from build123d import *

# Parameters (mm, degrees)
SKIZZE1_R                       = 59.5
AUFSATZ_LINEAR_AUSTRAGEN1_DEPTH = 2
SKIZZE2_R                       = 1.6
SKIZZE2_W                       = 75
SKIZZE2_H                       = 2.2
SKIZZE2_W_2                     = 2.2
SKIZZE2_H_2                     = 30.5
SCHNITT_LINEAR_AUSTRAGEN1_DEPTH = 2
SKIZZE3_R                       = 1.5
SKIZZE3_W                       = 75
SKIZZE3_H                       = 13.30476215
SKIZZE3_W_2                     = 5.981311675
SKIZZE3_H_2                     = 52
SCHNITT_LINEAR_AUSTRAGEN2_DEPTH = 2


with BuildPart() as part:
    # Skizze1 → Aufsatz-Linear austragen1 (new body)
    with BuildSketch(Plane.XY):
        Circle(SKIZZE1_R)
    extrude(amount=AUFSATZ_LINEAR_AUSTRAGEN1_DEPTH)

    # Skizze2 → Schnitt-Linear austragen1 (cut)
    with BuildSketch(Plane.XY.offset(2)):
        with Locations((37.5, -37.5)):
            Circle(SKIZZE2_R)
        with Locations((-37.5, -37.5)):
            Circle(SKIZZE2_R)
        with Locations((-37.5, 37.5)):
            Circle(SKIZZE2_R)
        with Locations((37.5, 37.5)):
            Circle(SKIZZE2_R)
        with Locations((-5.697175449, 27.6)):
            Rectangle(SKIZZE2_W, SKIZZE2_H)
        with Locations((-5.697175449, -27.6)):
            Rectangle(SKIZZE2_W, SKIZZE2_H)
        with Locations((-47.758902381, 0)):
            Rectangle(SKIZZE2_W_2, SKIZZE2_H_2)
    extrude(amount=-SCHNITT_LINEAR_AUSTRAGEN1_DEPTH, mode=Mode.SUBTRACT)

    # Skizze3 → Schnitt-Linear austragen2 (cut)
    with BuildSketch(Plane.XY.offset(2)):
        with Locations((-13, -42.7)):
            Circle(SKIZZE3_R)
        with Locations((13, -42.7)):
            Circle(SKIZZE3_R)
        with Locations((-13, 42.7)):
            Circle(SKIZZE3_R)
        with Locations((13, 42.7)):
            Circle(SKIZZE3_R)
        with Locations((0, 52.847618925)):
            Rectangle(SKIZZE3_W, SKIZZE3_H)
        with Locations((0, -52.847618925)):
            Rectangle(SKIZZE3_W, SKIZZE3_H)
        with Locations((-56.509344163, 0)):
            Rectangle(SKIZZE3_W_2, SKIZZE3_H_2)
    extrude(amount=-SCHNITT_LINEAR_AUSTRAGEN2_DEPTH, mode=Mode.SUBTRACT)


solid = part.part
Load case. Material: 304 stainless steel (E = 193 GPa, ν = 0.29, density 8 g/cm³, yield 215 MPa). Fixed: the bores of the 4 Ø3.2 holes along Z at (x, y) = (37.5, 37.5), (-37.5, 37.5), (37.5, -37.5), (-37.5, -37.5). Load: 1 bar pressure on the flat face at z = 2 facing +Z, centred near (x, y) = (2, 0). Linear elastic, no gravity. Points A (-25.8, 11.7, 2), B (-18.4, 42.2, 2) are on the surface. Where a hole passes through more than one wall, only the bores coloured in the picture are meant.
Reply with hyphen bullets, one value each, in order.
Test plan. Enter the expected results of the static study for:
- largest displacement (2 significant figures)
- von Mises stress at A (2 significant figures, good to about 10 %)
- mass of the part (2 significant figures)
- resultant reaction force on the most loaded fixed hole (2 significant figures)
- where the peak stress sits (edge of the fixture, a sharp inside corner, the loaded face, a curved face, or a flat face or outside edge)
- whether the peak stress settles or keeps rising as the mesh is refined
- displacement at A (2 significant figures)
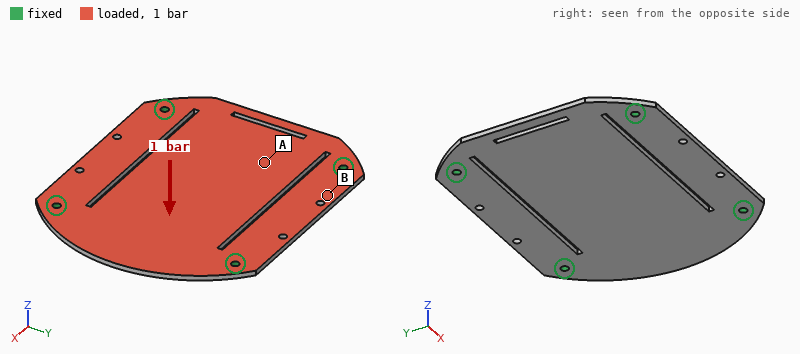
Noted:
- 0.28 mm
- 44 MPa
- 150 g
- 250 N
- edge of the fixture
- keeps rising
- 0.22 mm
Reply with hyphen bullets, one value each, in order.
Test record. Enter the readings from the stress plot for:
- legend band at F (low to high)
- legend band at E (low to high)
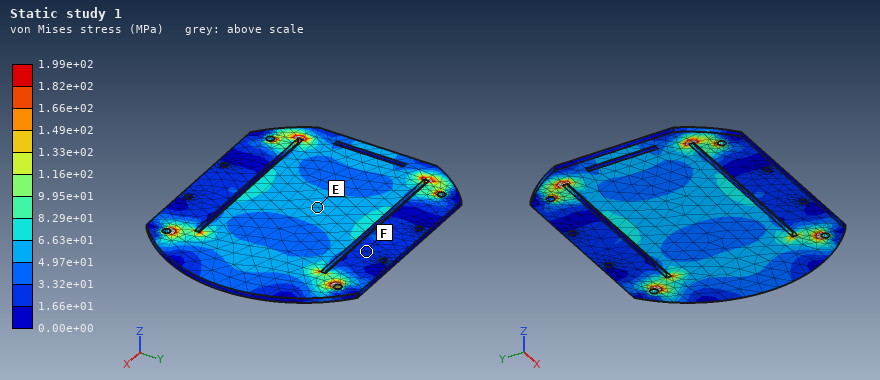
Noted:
- 1.66e+01 to 3.32e+01 MPa
- 4.97e+01 to 6.63e+01 MPa
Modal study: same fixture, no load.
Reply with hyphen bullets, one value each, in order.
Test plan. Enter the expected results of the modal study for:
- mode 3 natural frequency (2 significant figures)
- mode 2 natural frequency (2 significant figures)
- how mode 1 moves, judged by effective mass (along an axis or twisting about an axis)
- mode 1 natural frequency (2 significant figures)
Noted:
- 1600 Hz
- 1500 Hz
- along Z
- 850 Hz
